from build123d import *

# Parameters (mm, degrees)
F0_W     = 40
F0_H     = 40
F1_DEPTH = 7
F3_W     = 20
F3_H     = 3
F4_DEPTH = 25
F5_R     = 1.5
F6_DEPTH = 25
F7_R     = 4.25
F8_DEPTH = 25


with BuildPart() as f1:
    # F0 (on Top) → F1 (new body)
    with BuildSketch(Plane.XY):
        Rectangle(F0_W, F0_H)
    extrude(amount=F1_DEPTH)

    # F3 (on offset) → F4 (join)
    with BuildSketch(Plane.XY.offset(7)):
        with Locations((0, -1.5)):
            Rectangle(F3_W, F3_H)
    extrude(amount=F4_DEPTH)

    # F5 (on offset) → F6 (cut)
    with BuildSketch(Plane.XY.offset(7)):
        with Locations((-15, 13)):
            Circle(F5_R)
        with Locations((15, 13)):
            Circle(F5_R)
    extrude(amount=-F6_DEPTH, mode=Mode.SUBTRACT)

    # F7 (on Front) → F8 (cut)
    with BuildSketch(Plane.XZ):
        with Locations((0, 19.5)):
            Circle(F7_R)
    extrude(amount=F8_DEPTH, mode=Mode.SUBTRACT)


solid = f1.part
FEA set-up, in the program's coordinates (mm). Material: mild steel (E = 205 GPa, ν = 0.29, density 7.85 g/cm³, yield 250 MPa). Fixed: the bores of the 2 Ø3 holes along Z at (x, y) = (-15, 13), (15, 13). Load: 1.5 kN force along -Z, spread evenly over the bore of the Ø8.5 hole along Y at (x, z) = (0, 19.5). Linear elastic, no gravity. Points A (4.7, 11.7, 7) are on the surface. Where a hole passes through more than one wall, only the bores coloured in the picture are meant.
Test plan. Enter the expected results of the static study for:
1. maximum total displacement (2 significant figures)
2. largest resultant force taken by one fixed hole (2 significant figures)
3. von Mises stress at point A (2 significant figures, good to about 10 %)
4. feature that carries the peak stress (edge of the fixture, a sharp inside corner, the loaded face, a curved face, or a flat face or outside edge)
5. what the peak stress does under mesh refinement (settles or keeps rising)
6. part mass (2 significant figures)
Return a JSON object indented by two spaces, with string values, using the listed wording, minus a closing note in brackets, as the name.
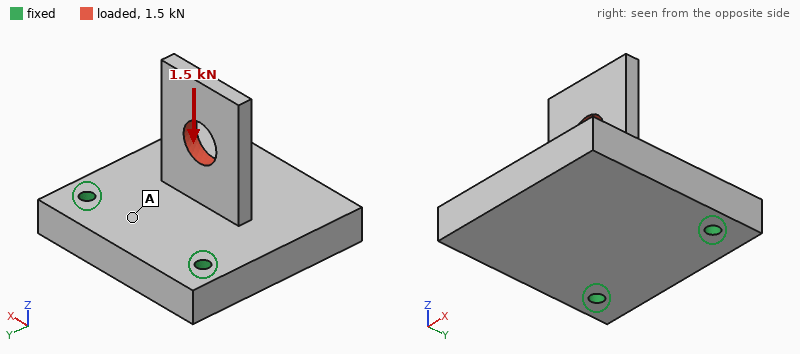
{
  "maximum total displacement": "34 µm",
  "largest resultant force taken by one fixed hole": "750 N",
  "von Mises stress at point A": "26 MPa",
  "feature that carries the peak stress": "edge of the fixture",
  "what the peak stress does under mesh refinement": "keeps rising",
  "part mass": "98 g"
}
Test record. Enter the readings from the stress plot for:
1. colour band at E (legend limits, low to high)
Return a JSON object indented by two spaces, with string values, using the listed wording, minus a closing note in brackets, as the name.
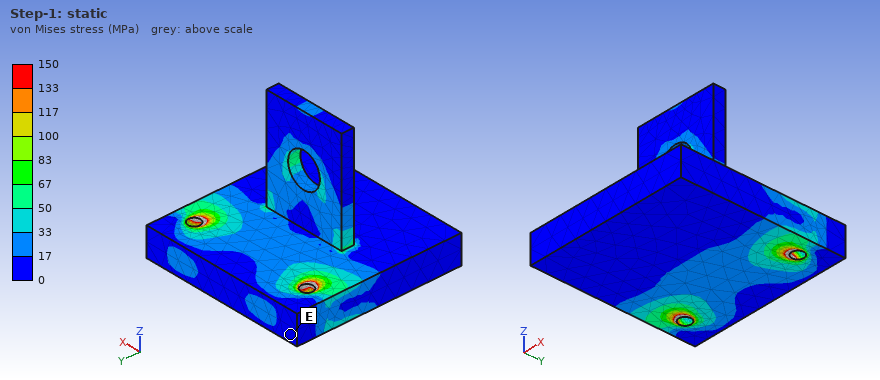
{
  "colour band at E": "0 to 17 MPa"
}
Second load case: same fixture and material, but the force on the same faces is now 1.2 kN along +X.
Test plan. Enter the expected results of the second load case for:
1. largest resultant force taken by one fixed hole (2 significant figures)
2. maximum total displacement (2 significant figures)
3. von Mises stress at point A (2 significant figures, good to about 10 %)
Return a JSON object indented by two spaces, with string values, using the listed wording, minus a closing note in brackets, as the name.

{
  "largest resultant force taken by one fixed hole": "1.0 kN",
  "maximum total displacement": "27 µm",
  "von Mises stress at point A": "20 MPa"
}
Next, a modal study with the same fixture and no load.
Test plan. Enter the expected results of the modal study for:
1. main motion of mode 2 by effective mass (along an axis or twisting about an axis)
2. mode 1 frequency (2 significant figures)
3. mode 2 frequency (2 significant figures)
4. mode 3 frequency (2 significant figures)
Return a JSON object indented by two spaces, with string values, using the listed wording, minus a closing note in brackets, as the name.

{
  "main motion of mode 2 by effective mass": "along Z",
  "mode 1 frequency": "3200 Hz",
  "mode 2 frequency": "4700 Hz",
  "mode 3 frequency": "8800 Hz"
}
